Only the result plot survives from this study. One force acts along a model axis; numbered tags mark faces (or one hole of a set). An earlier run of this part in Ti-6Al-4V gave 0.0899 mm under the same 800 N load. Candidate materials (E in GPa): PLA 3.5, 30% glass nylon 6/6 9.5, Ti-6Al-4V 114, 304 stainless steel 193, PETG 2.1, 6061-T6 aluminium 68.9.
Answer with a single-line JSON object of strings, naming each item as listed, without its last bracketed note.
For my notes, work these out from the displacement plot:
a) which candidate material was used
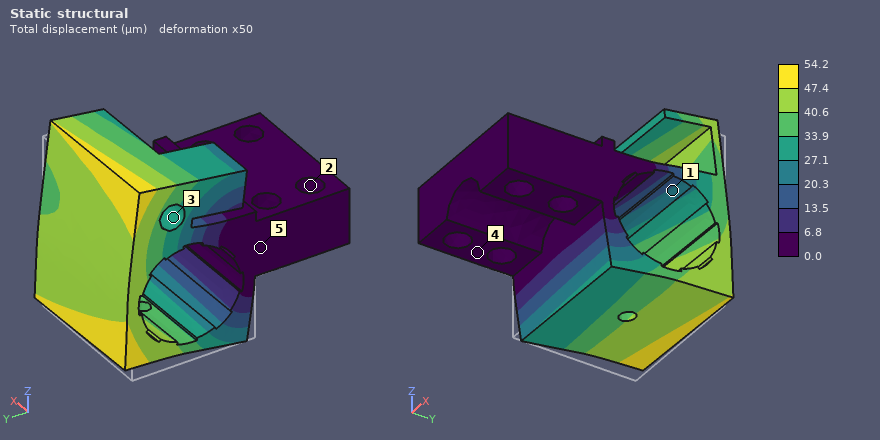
{"which candidate material was used": "304 stainless steel"}
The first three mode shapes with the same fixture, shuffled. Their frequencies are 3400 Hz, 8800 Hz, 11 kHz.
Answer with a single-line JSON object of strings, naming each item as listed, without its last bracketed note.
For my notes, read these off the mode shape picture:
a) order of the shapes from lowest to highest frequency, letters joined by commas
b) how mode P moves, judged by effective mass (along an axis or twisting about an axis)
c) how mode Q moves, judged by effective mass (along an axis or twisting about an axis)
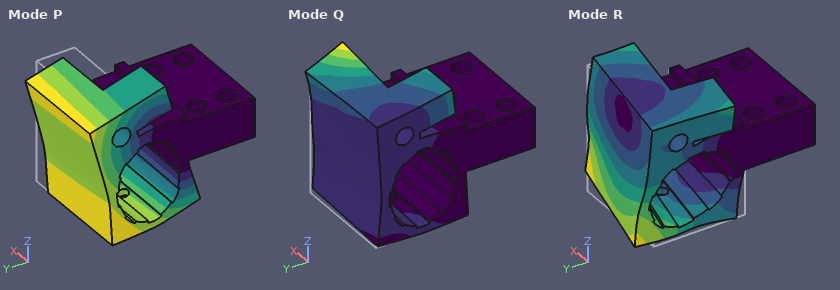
{"order of the shapes from lowest to highest frequency, letters joined by commas": "P, R, Q", "how mode P moves, judged by effective mass": "along Z", "how mode Q moves, judged by effective mass": "along Z"}
